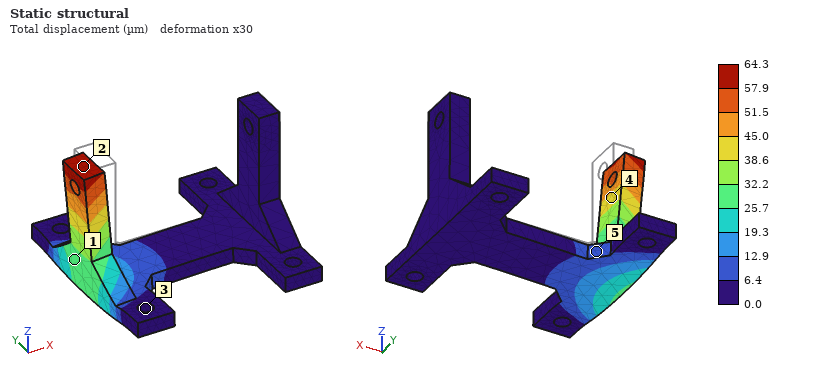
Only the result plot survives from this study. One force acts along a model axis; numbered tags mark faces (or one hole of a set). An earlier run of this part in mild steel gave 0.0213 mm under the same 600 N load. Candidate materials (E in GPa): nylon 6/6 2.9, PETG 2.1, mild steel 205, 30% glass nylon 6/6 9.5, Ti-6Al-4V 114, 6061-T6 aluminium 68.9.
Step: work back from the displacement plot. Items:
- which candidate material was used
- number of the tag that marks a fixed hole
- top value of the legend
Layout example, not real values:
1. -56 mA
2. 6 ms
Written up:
1. 6061-T6 aluminium
2. 3
3. 64.3 µm
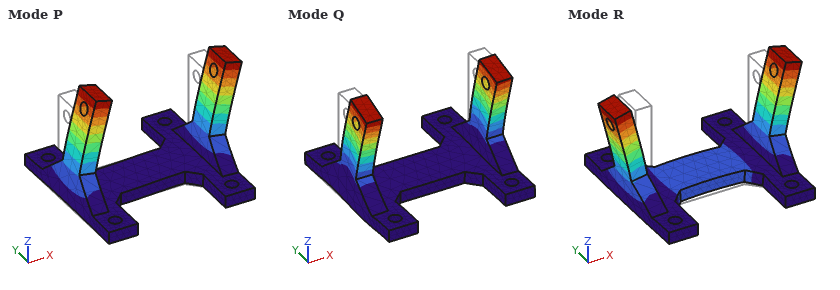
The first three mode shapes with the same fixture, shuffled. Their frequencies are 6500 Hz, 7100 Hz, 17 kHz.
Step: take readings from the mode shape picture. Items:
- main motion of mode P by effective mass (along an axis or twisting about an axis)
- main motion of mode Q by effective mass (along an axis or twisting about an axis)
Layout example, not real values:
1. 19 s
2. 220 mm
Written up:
1. along X
2. along Y
